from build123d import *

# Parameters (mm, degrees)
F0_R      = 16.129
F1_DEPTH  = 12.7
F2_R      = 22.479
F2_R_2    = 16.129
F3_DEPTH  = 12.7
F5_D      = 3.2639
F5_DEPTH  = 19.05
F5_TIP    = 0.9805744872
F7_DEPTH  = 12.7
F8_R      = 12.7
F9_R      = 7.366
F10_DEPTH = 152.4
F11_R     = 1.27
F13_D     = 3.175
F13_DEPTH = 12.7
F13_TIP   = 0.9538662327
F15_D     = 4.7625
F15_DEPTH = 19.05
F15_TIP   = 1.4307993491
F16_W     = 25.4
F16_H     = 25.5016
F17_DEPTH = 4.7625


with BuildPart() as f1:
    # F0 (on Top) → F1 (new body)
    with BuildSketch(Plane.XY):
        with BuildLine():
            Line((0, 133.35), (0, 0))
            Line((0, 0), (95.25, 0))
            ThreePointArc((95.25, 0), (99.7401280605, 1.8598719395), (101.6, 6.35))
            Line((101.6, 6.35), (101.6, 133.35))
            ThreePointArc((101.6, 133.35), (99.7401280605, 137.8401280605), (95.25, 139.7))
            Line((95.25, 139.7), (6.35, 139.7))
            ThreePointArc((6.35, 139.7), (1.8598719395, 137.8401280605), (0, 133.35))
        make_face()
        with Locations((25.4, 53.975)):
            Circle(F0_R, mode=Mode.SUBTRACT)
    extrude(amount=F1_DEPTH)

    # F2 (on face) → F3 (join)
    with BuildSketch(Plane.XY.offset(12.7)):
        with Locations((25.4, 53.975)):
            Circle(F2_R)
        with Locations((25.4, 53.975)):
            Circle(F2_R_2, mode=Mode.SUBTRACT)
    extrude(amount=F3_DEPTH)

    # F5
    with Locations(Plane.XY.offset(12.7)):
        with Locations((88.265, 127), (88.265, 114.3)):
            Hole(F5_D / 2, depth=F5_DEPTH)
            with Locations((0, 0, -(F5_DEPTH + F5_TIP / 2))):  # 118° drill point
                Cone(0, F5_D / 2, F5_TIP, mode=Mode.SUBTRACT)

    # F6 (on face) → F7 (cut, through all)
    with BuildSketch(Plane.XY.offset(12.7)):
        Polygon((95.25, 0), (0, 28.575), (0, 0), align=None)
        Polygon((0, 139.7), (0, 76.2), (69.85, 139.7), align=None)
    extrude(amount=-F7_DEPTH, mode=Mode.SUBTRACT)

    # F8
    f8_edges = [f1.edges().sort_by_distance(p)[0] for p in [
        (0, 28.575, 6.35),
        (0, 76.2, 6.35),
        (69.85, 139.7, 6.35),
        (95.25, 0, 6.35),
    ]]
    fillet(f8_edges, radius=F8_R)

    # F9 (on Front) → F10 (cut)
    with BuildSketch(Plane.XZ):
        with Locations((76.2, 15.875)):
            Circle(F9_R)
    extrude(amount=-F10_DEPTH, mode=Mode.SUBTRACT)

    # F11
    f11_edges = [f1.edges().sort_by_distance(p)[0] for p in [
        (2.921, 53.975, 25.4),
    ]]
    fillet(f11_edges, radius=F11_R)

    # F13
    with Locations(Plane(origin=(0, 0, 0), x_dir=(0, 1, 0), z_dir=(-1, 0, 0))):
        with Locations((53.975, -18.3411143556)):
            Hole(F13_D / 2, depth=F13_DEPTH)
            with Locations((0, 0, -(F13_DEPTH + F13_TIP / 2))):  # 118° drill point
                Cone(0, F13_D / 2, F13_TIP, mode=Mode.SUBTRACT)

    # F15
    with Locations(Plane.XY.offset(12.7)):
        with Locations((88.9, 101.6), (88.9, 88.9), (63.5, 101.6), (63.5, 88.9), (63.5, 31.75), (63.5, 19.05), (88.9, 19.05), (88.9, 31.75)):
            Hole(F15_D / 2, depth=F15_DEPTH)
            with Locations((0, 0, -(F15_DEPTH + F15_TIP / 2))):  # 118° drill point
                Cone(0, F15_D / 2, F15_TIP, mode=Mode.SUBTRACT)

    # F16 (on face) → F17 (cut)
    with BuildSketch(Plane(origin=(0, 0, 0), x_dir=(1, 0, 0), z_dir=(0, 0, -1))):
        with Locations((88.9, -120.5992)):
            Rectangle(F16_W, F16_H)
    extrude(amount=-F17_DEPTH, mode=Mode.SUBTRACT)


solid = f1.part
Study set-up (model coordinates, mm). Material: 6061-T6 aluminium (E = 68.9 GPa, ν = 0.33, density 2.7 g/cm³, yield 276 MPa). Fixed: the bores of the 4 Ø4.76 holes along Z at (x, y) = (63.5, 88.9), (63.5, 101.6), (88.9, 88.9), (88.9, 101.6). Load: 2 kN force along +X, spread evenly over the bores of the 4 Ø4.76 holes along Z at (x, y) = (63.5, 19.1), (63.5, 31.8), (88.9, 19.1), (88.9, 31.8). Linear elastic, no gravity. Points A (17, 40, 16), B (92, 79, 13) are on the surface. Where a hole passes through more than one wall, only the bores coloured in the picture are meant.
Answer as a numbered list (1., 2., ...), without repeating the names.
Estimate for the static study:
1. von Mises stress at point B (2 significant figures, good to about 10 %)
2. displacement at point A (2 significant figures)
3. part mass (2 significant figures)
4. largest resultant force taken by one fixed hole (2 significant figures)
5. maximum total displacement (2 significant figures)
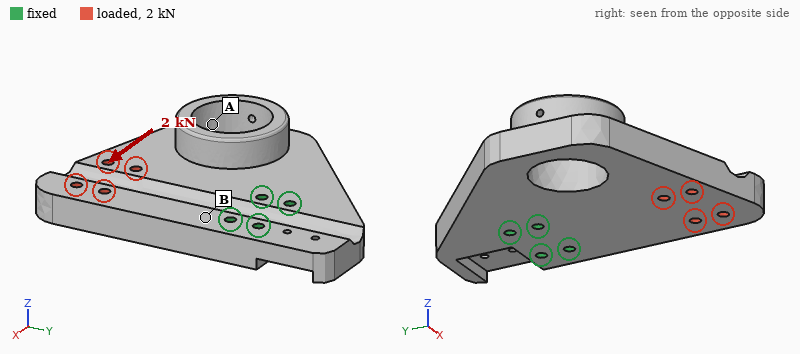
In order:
1. 11 MPa
2. 25 µm
3. 330 g
4. 3.1 kN
5. 34 µm
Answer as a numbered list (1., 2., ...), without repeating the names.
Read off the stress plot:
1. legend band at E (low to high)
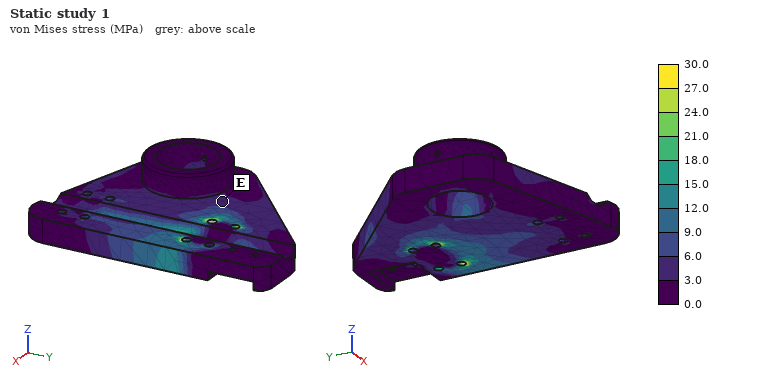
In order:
1. 3.0 to 6.0 MPa
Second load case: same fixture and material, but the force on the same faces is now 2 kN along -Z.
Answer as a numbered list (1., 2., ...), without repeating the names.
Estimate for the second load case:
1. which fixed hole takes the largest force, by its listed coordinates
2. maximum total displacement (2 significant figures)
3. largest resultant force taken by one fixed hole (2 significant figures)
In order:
1. (63.5, 88.9)
2. 0.38 mm
3. 3.0 kN
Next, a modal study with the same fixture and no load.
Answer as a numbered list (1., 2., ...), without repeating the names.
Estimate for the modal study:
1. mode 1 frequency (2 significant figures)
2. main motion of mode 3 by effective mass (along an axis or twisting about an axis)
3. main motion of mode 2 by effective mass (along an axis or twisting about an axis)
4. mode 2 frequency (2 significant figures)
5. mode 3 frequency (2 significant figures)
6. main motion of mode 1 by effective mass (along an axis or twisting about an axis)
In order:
1. 1300 Hz
2. along X
3. twisting about Y
4. 2100 Hz
5. 3500 Hz
6. along Z
